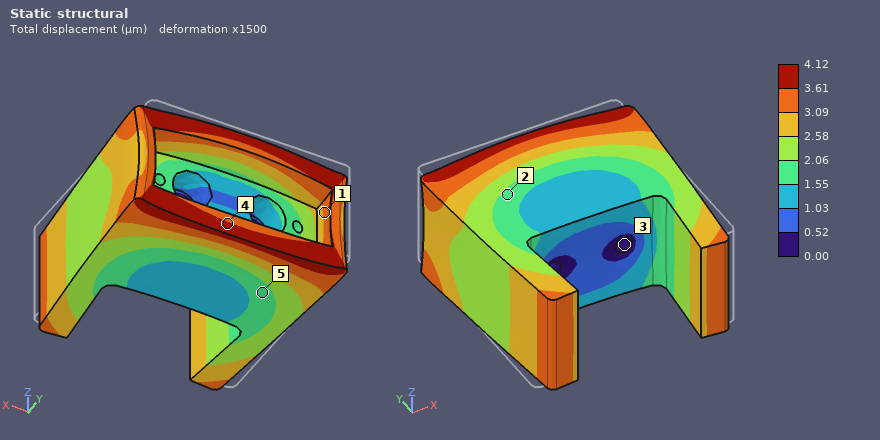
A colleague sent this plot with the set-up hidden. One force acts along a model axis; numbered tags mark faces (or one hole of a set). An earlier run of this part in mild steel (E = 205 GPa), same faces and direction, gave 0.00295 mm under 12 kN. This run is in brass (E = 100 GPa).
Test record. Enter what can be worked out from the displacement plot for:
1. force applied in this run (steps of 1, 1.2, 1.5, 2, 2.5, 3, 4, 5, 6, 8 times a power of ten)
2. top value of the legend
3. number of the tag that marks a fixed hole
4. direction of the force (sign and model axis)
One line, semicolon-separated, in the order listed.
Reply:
8 kN; 4.12 µm; 3; -Y
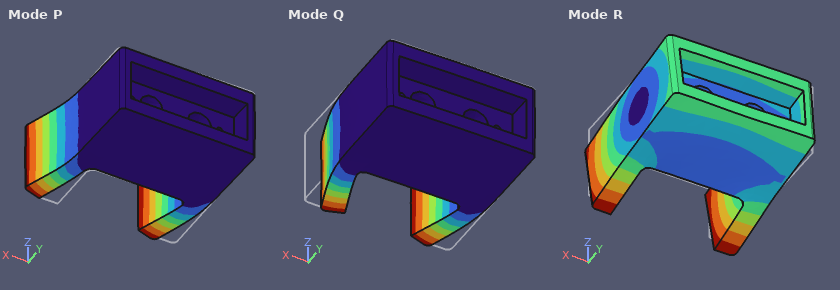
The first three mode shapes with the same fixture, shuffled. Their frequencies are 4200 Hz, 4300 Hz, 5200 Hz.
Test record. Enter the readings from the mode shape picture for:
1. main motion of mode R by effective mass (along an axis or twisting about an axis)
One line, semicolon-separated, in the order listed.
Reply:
twisting about X
